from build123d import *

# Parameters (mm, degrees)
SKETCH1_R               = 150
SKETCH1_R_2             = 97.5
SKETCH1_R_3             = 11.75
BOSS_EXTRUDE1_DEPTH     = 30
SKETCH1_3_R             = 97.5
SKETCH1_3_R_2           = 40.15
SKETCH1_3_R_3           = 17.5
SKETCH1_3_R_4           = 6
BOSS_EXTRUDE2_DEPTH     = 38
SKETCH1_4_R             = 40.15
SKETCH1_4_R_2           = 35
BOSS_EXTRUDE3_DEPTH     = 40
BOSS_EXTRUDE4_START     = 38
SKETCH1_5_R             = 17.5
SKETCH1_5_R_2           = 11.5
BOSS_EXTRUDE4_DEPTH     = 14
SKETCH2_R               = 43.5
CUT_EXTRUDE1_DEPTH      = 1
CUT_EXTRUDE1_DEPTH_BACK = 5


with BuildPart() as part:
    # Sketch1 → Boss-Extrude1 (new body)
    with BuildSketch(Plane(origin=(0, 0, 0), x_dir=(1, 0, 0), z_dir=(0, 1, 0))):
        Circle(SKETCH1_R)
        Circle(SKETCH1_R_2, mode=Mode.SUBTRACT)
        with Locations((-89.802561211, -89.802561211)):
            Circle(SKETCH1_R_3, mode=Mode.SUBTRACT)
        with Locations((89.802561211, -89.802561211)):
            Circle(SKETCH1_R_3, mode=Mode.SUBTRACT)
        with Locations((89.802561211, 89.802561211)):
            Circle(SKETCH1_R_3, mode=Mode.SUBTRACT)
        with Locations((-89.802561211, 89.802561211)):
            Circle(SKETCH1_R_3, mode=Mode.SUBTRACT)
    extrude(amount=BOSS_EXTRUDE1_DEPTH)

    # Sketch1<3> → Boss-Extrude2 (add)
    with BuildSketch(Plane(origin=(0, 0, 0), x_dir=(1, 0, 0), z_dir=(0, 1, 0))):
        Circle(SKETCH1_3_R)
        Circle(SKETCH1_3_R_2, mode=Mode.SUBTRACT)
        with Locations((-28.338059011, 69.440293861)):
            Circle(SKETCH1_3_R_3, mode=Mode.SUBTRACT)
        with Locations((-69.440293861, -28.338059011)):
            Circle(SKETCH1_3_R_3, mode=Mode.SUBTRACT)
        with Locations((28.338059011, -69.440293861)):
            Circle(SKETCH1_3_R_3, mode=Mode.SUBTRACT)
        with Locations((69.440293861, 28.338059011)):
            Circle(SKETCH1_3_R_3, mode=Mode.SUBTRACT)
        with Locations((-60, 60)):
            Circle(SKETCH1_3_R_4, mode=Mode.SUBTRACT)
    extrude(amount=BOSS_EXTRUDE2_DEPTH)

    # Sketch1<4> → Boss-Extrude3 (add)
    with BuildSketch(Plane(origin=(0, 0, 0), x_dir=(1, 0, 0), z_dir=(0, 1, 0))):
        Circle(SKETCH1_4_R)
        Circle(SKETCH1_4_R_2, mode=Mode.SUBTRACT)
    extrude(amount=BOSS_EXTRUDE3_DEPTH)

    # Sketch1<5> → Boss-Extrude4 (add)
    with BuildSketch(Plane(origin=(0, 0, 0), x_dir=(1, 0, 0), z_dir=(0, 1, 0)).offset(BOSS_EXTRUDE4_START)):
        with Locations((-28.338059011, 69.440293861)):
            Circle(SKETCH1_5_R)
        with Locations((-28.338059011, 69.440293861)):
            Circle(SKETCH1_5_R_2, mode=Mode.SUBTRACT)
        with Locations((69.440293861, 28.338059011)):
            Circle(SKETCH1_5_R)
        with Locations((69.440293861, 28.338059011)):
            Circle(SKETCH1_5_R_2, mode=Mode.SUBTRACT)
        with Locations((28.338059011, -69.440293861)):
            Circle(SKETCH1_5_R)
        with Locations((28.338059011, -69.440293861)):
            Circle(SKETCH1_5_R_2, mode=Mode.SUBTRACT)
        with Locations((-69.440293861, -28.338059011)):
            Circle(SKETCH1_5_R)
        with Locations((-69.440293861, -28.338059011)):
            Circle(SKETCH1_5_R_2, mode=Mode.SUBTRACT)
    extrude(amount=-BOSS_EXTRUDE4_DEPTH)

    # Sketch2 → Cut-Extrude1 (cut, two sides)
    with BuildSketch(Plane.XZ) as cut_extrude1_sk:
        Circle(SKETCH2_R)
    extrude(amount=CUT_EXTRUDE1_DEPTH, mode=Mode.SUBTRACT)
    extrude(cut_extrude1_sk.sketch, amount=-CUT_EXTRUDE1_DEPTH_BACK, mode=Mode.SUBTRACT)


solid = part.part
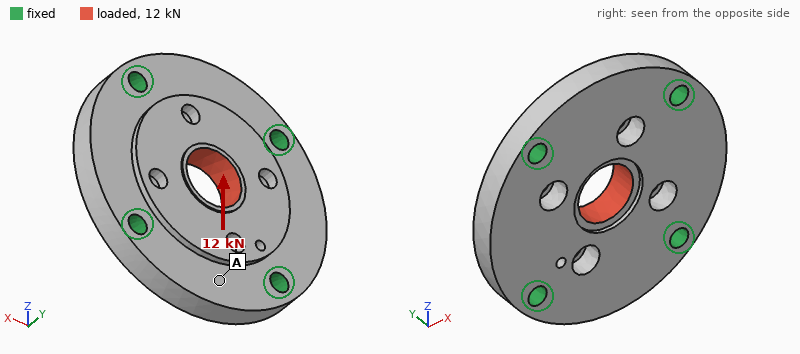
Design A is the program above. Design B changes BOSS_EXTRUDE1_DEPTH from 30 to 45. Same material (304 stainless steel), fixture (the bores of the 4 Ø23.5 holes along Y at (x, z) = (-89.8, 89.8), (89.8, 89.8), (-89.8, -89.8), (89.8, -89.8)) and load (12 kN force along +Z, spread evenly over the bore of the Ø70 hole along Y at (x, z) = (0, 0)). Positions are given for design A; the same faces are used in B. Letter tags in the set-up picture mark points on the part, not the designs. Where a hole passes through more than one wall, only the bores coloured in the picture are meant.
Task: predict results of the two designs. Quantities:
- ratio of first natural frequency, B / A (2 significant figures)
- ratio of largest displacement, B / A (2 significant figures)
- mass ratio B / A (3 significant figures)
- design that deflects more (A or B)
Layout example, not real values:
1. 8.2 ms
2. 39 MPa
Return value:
1. 1.3
2. 0.84
3. 1.29
4. A
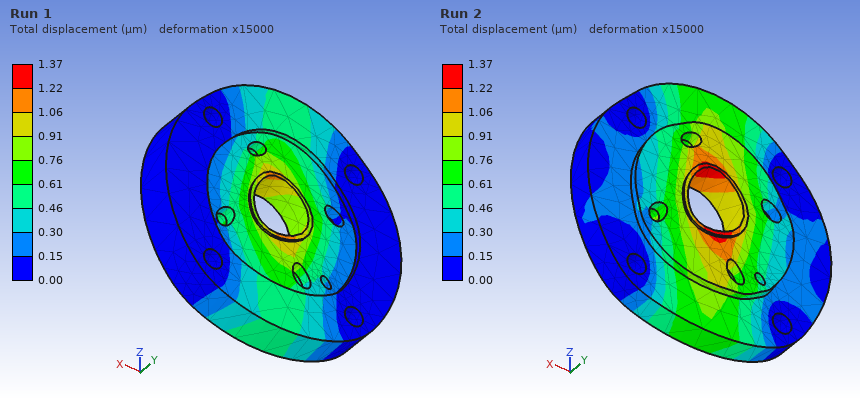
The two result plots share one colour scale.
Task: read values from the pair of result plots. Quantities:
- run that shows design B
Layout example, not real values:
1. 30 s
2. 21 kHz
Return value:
1. Run 1
